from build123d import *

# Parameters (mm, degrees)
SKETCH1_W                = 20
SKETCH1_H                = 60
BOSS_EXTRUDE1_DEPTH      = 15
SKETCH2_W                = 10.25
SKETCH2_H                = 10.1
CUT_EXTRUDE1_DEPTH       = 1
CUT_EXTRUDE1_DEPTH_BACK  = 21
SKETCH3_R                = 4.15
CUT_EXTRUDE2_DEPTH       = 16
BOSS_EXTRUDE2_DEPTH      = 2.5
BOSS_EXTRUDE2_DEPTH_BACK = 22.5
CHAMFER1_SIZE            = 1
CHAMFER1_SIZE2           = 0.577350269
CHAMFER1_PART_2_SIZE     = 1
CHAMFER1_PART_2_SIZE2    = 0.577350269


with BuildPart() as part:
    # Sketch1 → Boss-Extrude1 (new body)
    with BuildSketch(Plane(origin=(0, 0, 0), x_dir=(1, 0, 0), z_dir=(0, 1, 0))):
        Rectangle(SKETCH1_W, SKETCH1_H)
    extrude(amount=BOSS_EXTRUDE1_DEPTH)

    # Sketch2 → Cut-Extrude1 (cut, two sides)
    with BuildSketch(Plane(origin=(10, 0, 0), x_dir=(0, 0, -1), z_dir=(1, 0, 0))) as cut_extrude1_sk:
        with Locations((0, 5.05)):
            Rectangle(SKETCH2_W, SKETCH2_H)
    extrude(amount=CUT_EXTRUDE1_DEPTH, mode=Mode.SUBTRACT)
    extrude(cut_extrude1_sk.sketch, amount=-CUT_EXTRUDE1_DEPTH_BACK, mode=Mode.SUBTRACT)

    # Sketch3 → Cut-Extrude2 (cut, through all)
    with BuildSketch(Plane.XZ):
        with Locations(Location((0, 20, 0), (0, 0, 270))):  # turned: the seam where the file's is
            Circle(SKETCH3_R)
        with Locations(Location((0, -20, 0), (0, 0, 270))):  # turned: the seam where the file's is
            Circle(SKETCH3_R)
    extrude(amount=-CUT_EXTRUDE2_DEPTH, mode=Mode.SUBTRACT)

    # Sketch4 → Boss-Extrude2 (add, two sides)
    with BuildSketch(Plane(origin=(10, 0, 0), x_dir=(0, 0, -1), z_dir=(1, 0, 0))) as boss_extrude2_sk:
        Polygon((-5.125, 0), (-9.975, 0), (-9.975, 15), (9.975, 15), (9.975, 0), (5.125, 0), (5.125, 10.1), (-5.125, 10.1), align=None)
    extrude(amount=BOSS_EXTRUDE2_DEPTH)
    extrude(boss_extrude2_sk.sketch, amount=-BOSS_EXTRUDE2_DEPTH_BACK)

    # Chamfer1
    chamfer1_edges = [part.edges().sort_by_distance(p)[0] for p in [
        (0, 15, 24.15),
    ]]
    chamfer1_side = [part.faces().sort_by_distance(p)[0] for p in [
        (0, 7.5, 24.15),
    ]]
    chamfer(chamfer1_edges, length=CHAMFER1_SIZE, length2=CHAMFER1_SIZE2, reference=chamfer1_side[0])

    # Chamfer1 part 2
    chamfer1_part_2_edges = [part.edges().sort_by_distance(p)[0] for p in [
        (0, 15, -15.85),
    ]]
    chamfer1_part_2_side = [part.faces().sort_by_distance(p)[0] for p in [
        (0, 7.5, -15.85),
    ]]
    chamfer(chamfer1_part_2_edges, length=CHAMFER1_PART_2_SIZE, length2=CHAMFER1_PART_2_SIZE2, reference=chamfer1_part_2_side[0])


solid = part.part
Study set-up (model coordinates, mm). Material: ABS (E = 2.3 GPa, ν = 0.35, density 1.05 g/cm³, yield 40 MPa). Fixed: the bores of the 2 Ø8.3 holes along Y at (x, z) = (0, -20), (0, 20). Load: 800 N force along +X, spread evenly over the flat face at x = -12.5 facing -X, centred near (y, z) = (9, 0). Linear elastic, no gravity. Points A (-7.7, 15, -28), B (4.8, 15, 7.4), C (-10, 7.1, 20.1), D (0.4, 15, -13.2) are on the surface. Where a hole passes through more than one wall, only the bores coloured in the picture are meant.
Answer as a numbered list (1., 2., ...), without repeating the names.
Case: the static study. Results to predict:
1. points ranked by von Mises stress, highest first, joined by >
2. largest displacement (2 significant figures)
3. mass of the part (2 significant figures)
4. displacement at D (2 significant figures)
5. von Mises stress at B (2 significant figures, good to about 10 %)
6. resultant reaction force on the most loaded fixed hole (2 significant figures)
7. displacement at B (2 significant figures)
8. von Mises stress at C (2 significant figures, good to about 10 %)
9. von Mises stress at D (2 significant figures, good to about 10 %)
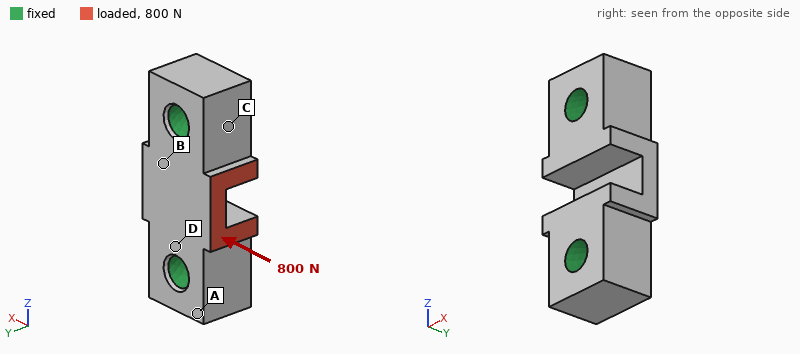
1. D > B > C > A
2. 62 µm
3. 16 g
4. 14 µm
5. 2.9 MPa
6. 400 N
7. 30 µm
8. 1.7 MPa
9. 4.4 MPa
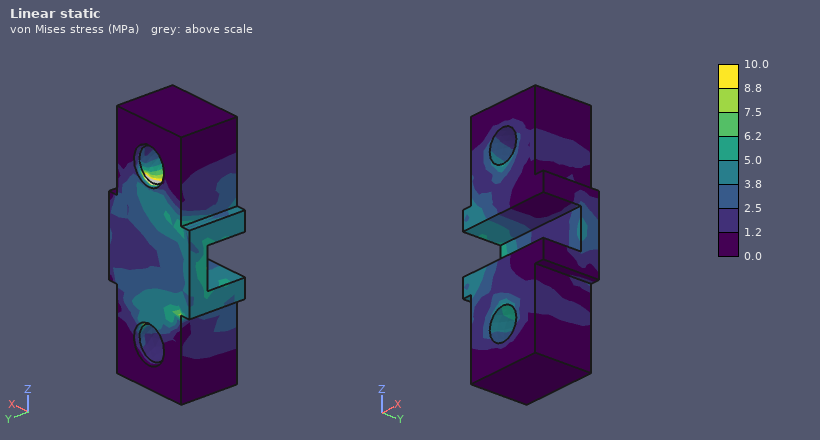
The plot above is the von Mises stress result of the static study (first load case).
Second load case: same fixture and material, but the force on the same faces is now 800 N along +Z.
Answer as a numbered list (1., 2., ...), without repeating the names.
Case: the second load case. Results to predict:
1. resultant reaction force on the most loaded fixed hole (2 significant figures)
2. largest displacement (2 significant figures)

1. 450 N
2. 89 µm
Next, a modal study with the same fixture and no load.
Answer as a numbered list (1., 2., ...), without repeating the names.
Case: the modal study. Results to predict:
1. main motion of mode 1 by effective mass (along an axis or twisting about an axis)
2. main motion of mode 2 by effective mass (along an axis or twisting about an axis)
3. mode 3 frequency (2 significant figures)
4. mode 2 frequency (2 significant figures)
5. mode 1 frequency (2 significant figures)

1. along X
2. along Y
3. 11 kHz
4. 10000 Hz
5. 9200 Hz
